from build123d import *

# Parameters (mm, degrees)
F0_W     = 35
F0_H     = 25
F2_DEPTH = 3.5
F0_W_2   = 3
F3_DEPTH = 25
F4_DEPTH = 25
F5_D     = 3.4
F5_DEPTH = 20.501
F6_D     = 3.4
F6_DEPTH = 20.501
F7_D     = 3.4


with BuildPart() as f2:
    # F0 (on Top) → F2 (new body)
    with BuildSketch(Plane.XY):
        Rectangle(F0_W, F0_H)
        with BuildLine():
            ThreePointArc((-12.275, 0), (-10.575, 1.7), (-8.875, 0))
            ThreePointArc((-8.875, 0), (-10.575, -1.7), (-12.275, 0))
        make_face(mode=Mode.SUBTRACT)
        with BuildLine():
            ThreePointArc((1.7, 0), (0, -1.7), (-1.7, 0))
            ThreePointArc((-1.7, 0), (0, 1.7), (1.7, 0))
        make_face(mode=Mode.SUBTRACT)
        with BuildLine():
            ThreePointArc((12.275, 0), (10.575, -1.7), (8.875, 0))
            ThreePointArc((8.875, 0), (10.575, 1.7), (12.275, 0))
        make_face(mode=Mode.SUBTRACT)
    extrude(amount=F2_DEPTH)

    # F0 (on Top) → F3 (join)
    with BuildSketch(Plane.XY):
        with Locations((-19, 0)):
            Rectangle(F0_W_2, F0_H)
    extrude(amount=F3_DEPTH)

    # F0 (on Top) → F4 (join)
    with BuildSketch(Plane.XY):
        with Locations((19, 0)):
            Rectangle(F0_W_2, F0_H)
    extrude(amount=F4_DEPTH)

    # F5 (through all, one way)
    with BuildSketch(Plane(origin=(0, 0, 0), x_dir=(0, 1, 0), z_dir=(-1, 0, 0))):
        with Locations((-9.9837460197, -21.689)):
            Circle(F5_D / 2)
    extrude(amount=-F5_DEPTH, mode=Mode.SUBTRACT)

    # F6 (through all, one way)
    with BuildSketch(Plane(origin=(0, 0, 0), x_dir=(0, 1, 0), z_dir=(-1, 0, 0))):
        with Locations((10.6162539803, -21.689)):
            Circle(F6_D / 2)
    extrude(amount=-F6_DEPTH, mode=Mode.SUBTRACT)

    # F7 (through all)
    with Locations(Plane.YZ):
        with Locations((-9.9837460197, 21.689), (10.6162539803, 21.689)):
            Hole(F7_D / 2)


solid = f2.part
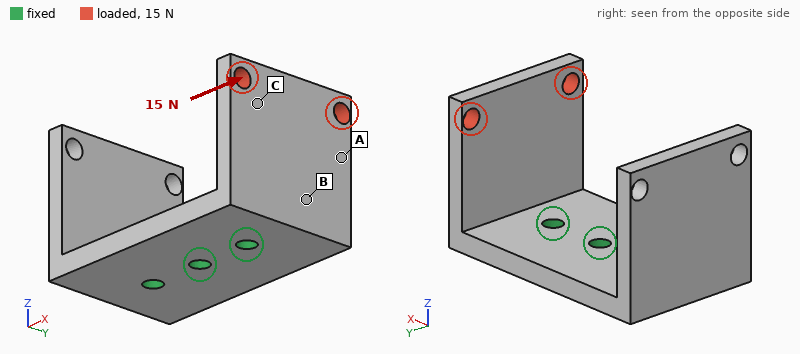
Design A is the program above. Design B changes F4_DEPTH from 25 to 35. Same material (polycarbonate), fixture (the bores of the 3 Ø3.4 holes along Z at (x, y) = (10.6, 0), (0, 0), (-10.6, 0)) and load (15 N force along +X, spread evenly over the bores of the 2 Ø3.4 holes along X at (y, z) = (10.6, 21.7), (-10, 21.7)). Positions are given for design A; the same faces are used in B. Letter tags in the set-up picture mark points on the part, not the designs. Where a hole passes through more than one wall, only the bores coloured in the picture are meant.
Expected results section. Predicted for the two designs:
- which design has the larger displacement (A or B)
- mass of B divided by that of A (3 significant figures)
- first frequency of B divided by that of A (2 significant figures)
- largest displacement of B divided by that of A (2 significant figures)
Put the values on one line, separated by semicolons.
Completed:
B; 1.11; 0.52; 1.5
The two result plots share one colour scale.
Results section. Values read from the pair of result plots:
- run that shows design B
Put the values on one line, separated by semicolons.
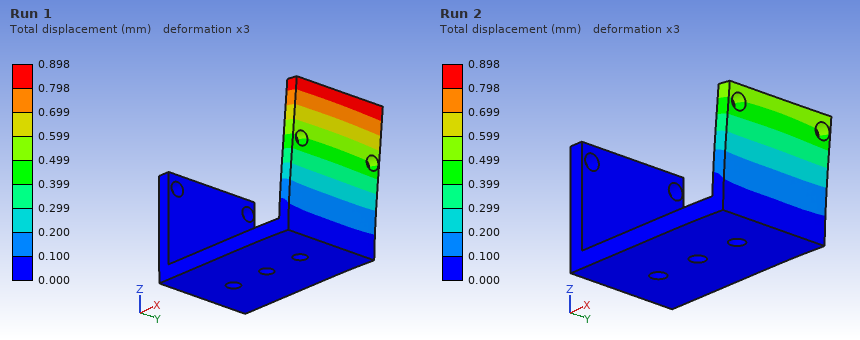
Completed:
Run 1
